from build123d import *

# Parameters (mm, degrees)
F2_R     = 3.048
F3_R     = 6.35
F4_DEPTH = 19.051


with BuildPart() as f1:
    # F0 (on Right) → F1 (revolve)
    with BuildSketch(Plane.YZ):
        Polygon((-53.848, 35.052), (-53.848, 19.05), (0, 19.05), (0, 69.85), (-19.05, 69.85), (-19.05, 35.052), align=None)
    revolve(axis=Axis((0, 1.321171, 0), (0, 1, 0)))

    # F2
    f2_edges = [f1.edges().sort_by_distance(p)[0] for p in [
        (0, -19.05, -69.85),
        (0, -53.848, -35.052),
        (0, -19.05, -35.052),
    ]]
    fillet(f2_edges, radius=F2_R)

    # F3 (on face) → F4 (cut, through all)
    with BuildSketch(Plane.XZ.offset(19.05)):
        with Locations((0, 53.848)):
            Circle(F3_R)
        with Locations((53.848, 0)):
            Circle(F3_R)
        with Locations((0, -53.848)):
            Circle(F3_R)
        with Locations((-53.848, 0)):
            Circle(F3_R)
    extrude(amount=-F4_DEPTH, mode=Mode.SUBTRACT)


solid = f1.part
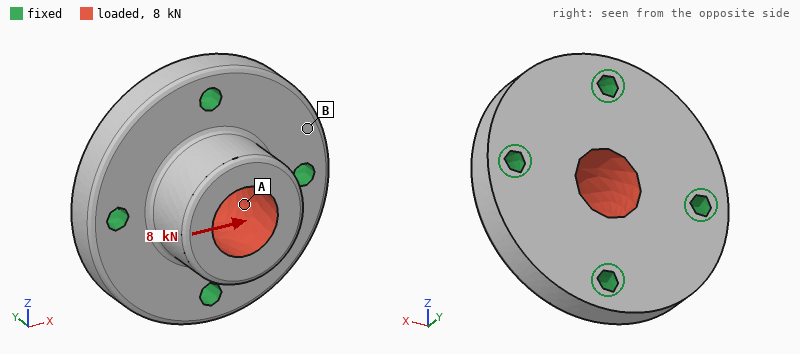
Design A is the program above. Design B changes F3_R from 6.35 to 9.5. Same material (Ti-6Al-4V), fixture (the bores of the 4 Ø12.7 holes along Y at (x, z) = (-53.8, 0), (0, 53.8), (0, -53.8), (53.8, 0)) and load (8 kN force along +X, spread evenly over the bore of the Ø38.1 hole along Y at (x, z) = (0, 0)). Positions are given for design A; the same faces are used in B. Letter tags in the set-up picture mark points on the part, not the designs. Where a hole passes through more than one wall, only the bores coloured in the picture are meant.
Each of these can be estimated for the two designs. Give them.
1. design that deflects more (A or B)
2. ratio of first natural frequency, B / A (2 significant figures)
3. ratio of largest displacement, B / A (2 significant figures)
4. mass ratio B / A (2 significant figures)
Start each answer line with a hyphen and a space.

- A
- 1.1
- 0.88
- 0.97
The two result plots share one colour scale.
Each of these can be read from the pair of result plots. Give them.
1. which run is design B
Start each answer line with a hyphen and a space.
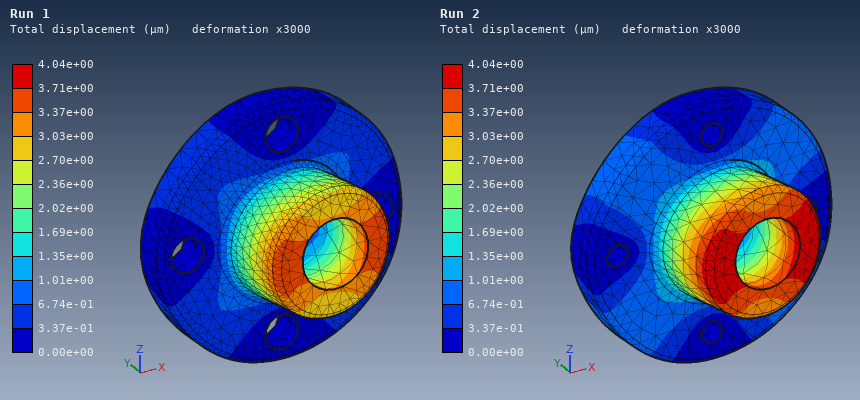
- Run 1
